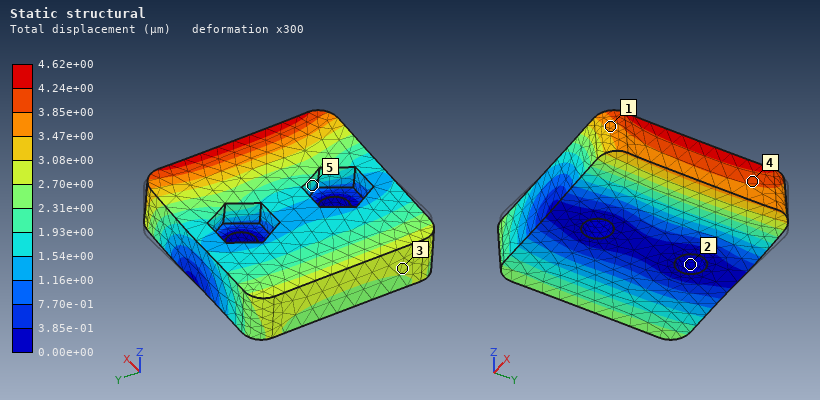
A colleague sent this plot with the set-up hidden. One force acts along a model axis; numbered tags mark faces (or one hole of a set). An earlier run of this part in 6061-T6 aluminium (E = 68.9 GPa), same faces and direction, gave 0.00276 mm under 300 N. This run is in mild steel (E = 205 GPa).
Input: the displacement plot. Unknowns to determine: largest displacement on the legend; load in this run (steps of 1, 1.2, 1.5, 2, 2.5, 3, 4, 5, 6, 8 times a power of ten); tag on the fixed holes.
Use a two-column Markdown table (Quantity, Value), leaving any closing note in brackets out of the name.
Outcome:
| Quantity | Value |
|---|---|
| largest displacement on the legend | 4.62e+00 µm |
| load in this run | 1.5 kN |
| tag on the fixed holes | 2 |
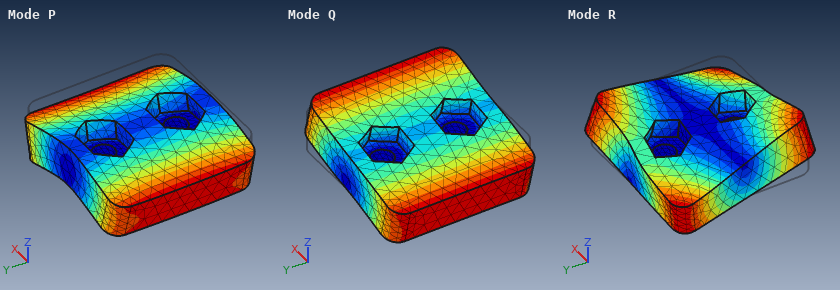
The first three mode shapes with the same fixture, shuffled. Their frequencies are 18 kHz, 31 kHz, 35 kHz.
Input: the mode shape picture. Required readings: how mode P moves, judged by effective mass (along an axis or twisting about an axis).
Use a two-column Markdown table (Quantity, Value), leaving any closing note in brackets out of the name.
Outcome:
| Quantity | Value |
|---|---|
| how mode P moves, judged by effective mass | along Z |
